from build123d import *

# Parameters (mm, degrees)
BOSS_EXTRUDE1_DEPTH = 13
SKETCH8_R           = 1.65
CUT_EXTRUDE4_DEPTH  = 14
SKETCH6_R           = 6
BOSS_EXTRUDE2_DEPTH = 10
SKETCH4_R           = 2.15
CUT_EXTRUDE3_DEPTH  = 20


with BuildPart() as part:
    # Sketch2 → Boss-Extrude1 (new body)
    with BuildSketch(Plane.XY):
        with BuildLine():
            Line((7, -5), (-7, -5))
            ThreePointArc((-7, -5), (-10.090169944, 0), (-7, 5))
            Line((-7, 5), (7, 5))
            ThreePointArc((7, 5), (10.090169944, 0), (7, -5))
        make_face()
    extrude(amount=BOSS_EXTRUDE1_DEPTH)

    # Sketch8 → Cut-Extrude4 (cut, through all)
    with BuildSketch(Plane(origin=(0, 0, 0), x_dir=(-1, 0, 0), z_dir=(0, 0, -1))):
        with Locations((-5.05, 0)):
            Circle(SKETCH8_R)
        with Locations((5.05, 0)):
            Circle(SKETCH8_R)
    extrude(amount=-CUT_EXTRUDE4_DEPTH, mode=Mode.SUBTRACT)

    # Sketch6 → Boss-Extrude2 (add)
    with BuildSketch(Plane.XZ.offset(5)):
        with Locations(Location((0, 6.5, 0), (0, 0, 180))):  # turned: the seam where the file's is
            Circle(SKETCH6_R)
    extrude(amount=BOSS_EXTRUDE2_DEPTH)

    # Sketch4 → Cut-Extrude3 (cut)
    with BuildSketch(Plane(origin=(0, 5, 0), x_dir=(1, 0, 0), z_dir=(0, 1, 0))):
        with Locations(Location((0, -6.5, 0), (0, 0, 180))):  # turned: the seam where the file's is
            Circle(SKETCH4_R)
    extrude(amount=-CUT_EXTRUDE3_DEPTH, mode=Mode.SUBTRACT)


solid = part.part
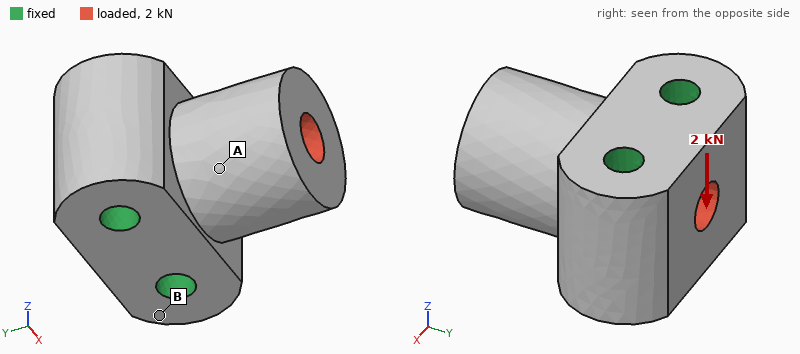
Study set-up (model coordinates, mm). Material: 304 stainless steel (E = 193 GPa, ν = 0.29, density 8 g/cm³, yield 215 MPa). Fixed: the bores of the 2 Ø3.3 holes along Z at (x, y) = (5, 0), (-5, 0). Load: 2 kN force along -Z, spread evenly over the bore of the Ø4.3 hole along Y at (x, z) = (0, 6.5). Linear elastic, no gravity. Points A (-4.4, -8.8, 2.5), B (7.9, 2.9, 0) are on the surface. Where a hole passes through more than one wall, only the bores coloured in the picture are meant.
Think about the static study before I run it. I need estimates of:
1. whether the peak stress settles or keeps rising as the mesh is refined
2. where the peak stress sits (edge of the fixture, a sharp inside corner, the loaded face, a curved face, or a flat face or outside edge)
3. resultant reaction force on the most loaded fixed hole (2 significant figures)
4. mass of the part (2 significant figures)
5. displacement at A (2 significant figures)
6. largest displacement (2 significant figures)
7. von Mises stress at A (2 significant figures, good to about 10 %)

keeps rising
edge of the fixture
1.0 kN
24 g
1.9 µm
3.5 µm
14 MPa
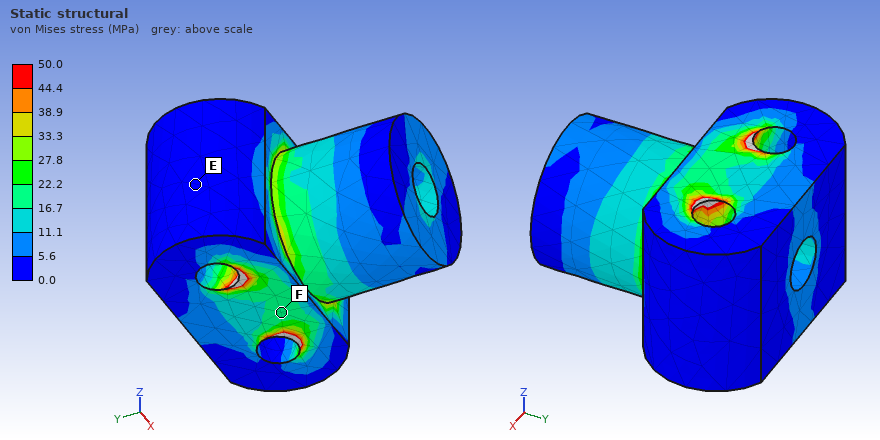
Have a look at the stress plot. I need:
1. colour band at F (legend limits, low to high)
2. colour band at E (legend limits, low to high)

16.7 to 22.2 MPa
0.0 to 5.6 MPa
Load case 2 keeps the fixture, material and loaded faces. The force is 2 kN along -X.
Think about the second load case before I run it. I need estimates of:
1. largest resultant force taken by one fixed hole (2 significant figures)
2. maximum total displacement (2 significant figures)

1.3 kN
2.7 µm
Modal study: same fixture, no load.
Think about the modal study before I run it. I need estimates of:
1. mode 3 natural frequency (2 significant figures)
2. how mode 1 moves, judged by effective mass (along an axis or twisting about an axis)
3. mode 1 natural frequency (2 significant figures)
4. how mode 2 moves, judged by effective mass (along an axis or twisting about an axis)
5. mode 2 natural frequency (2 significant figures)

63 kHz
along Z
36 kHz
along X
41 kHz
